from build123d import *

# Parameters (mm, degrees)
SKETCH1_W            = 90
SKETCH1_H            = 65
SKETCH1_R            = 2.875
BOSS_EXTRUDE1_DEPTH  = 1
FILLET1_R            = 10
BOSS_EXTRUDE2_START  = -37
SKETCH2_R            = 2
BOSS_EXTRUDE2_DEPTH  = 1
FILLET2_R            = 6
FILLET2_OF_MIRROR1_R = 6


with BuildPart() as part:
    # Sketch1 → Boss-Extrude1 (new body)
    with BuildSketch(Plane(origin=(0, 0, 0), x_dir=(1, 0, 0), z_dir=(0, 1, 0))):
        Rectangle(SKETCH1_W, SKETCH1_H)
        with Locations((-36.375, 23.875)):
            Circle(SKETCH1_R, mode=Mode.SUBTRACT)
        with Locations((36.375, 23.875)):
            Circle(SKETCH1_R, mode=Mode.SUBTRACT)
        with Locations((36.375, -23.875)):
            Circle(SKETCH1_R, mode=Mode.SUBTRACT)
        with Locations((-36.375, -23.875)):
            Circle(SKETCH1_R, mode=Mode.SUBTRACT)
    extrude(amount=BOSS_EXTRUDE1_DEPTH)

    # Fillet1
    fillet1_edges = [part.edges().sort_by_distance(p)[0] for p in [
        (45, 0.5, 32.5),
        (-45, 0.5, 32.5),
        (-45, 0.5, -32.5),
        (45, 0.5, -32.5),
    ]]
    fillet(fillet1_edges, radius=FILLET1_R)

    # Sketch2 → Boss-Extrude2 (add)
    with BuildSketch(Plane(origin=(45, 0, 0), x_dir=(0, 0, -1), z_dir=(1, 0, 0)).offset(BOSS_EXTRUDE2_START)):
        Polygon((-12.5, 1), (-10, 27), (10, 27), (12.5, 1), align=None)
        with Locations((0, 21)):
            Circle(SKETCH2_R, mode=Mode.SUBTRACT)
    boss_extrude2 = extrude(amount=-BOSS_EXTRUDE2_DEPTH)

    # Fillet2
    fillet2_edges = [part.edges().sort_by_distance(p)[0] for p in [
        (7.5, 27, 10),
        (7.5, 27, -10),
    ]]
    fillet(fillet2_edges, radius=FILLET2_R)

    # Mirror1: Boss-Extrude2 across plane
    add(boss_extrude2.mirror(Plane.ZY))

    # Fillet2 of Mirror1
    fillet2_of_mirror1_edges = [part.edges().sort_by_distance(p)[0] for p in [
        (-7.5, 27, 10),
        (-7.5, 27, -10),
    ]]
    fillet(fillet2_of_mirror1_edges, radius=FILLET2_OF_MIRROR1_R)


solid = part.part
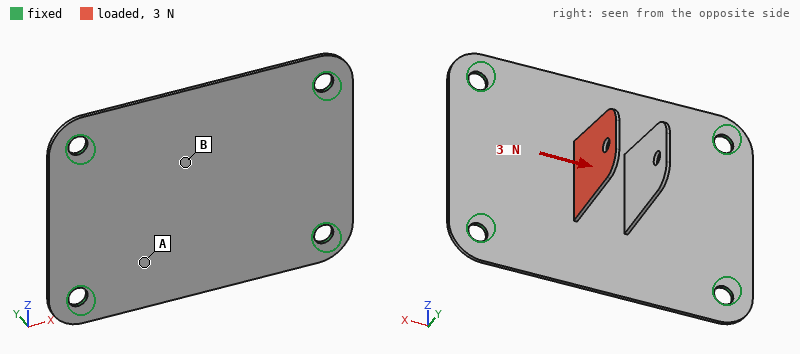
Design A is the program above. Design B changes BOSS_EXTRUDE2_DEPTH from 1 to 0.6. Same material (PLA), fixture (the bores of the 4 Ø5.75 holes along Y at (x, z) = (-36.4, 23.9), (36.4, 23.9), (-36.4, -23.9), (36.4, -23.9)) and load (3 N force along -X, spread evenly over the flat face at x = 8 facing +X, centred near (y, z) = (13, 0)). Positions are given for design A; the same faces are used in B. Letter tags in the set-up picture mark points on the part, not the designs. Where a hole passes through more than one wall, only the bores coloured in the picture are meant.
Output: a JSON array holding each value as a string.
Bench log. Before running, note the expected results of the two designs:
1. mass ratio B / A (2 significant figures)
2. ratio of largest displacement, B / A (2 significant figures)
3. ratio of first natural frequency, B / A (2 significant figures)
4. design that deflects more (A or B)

["0.93", "3.5", "0.99", "B"]
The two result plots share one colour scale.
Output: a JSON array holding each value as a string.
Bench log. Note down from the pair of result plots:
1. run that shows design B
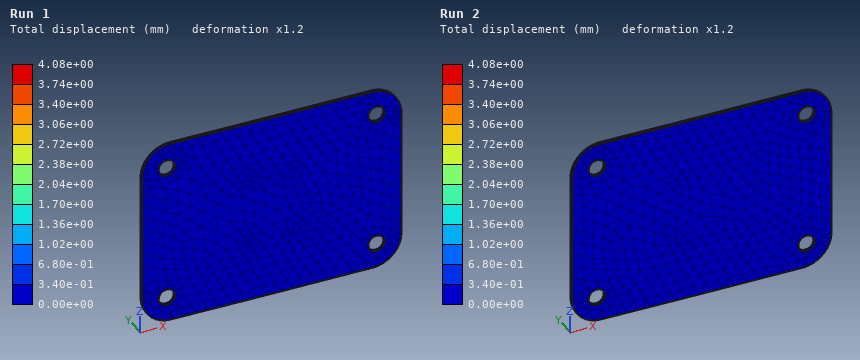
["Run 1"]
